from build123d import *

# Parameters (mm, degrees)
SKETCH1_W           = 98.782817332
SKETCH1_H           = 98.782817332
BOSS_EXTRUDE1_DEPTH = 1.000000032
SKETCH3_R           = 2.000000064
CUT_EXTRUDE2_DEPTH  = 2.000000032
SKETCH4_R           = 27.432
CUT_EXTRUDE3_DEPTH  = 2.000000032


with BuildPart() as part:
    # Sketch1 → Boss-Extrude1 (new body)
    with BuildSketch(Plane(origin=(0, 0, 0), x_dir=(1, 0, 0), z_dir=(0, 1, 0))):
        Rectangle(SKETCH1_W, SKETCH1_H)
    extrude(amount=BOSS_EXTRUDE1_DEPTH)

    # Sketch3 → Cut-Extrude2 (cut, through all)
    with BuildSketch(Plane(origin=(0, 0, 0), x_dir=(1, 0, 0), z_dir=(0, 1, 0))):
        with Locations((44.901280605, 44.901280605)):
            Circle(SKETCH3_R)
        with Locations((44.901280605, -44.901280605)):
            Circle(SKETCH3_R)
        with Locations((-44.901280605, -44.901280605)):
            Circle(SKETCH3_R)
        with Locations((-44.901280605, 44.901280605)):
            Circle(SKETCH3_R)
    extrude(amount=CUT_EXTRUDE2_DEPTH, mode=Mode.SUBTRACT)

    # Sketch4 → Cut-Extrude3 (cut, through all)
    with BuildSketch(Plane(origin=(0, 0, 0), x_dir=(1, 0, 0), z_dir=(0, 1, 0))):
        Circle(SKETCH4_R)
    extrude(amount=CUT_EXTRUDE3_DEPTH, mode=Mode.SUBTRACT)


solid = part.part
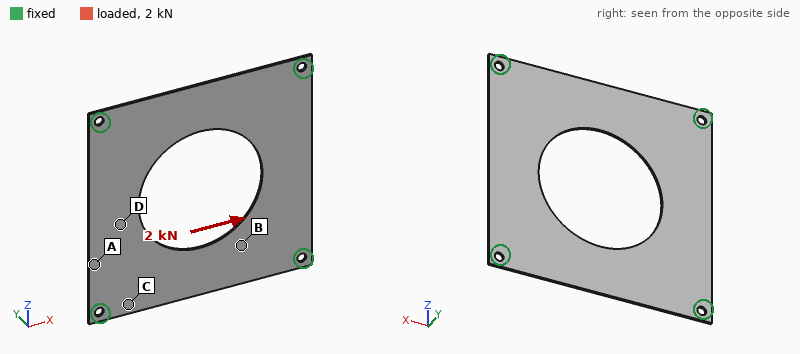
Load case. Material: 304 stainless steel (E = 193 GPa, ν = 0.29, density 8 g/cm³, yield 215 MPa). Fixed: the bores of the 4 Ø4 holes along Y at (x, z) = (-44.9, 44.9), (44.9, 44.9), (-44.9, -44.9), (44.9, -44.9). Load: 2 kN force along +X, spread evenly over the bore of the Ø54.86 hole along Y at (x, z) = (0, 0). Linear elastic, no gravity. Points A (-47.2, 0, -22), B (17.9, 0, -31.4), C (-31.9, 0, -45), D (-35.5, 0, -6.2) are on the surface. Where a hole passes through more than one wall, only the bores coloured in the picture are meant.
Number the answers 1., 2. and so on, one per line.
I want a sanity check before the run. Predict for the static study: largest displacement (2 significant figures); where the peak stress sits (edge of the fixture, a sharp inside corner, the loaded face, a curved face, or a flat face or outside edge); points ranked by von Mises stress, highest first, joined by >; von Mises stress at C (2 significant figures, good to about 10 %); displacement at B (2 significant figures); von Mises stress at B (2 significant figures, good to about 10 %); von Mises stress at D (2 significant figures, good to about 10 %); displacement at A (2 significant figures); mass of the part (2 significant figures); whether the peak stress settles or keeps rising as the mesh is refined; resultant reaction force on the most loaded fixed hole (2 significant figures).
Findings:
1. 11 µm
2. edge of the fixture
3. C > B > D > A
4. 29 MPa
5. 5.6 µm
6. 19 MPa
7. 11 MPa
8. 7.5 µm
9. 59 g
10. keeps rising
11. 550 N
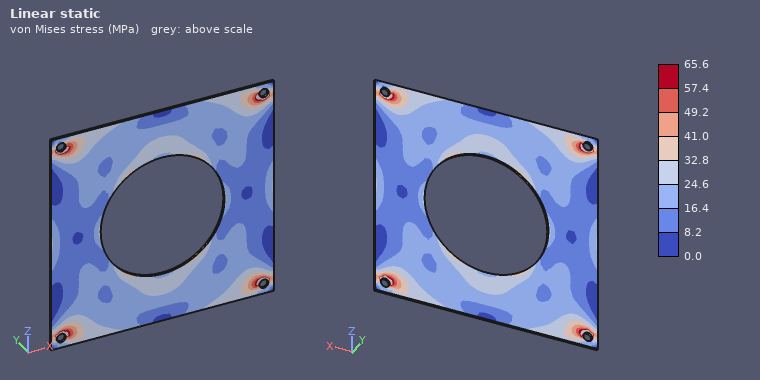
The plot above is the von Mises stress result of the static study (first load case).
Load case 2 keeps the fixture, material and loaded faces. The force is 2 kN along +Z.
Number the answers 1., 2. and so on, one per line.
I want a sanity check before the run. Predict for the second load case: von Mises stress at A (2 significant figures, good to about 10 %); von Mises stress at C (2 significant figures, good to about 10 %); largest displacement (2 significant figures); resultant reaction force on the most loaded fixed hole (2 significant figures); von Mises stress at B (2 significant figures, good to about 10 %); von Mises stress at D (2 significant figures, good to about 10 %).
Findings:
1. 25 MPa
2. 11 MPa
3. 11 µm
4. 550 N
5. 18 MPa
6. 25 MPa
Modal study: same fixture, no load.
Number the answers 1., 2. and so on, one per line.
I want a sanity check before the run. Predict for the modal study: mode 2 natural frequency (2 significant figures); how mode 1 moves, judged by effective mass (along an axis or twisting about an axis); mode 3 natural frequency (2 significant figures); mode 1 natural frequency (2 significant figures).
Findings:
1. 670 Hz
2. along Y
3. 670 Hz
4. 480 Hz
